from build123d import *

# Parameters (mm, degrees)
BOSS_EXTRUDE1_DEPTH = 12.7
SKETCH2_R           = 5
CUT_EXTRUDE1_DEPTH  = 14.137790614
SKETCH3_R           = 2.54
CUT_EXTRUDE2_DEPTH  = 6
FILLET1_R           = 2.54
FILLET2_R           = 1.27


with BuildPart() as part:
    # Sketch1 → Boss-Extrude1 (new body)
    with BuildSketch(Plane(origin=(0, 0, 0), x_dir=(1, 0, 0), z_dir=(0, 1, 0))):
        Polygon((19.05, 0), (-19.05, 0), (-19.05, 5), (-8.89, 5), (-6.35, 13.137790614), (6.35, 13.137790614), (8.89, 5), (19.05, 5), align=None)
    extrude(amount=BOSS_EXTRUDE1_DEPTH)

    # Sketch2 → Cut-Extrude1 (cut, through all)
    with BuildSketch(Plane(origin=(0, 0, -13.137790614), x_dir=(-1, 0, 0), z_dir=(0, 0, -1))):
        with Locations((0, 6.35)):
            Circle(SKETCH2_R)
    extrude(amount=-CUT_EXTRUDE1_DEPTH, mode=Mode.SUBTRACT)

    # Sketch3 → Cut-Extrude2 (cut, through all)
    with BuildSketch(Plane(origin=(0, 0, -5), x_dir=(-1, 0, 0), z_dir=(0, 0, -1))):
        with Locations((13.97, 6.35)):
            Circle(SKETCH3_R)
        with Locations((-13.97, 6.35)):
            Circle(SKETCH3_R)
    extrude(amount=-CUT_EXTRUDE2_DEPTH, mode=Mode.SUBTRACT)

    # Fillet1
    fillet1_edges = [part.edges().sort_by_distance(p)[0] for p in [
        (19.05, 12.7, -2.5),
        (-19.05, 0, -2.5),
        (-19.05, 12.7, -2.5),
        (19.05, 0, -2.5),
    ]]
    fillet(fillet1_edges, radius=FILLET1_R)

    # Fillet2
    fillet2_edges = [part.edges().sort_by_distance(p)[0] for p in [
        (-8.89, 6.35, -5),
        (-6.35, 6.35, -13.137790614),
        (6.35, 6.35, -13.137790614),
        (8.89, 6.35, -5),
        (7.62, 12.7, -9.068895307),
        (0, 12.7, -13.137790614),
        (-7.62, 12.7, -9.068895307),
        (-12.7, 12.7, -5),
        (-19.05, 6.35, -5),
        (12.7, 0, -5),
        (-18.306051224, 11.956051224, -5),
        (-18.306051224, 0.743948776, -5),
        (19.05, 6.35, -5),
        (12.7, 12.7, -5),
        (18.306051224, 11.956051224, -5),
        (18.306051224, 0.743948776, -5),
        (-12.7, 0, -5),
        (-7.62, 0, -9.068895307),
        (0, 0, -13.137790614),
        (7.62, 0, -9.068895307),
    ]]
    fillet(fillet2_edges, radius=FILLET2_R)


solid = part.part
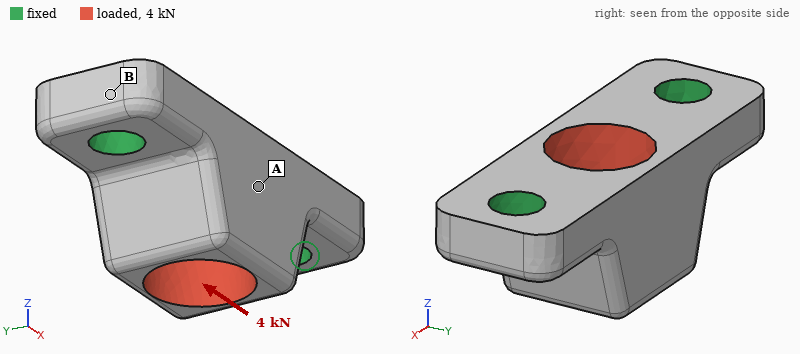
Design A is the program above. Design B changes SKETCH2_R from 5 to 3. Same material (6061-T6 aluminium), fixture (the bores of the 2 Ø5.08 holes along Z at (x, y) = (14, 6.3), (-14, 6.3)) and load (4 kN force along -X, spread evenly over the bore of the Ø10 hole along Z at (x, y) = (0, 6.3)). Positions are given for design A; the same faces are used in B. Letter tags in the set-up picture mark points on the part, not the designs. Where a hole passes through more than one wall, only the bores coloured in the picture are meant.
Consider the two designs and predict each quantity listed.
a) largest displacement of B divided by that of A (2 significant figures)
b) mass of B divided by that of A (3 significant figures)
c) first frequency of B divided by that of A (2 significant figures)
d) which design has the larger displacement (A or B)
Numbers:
0.71
1.25
0.86
A
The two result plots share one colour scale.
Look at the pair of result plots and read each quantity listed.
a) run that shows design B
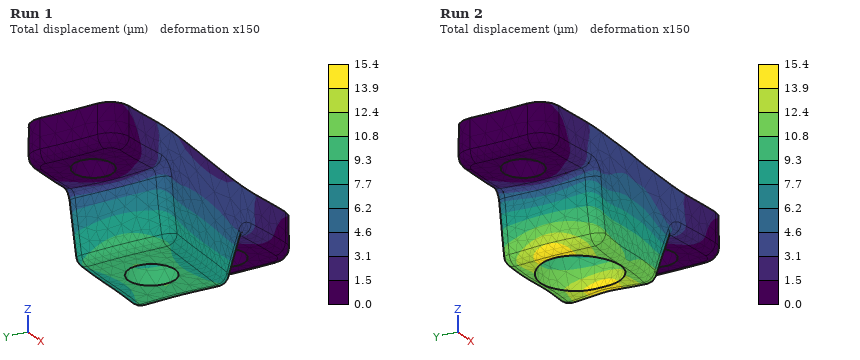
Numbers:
Run 1
